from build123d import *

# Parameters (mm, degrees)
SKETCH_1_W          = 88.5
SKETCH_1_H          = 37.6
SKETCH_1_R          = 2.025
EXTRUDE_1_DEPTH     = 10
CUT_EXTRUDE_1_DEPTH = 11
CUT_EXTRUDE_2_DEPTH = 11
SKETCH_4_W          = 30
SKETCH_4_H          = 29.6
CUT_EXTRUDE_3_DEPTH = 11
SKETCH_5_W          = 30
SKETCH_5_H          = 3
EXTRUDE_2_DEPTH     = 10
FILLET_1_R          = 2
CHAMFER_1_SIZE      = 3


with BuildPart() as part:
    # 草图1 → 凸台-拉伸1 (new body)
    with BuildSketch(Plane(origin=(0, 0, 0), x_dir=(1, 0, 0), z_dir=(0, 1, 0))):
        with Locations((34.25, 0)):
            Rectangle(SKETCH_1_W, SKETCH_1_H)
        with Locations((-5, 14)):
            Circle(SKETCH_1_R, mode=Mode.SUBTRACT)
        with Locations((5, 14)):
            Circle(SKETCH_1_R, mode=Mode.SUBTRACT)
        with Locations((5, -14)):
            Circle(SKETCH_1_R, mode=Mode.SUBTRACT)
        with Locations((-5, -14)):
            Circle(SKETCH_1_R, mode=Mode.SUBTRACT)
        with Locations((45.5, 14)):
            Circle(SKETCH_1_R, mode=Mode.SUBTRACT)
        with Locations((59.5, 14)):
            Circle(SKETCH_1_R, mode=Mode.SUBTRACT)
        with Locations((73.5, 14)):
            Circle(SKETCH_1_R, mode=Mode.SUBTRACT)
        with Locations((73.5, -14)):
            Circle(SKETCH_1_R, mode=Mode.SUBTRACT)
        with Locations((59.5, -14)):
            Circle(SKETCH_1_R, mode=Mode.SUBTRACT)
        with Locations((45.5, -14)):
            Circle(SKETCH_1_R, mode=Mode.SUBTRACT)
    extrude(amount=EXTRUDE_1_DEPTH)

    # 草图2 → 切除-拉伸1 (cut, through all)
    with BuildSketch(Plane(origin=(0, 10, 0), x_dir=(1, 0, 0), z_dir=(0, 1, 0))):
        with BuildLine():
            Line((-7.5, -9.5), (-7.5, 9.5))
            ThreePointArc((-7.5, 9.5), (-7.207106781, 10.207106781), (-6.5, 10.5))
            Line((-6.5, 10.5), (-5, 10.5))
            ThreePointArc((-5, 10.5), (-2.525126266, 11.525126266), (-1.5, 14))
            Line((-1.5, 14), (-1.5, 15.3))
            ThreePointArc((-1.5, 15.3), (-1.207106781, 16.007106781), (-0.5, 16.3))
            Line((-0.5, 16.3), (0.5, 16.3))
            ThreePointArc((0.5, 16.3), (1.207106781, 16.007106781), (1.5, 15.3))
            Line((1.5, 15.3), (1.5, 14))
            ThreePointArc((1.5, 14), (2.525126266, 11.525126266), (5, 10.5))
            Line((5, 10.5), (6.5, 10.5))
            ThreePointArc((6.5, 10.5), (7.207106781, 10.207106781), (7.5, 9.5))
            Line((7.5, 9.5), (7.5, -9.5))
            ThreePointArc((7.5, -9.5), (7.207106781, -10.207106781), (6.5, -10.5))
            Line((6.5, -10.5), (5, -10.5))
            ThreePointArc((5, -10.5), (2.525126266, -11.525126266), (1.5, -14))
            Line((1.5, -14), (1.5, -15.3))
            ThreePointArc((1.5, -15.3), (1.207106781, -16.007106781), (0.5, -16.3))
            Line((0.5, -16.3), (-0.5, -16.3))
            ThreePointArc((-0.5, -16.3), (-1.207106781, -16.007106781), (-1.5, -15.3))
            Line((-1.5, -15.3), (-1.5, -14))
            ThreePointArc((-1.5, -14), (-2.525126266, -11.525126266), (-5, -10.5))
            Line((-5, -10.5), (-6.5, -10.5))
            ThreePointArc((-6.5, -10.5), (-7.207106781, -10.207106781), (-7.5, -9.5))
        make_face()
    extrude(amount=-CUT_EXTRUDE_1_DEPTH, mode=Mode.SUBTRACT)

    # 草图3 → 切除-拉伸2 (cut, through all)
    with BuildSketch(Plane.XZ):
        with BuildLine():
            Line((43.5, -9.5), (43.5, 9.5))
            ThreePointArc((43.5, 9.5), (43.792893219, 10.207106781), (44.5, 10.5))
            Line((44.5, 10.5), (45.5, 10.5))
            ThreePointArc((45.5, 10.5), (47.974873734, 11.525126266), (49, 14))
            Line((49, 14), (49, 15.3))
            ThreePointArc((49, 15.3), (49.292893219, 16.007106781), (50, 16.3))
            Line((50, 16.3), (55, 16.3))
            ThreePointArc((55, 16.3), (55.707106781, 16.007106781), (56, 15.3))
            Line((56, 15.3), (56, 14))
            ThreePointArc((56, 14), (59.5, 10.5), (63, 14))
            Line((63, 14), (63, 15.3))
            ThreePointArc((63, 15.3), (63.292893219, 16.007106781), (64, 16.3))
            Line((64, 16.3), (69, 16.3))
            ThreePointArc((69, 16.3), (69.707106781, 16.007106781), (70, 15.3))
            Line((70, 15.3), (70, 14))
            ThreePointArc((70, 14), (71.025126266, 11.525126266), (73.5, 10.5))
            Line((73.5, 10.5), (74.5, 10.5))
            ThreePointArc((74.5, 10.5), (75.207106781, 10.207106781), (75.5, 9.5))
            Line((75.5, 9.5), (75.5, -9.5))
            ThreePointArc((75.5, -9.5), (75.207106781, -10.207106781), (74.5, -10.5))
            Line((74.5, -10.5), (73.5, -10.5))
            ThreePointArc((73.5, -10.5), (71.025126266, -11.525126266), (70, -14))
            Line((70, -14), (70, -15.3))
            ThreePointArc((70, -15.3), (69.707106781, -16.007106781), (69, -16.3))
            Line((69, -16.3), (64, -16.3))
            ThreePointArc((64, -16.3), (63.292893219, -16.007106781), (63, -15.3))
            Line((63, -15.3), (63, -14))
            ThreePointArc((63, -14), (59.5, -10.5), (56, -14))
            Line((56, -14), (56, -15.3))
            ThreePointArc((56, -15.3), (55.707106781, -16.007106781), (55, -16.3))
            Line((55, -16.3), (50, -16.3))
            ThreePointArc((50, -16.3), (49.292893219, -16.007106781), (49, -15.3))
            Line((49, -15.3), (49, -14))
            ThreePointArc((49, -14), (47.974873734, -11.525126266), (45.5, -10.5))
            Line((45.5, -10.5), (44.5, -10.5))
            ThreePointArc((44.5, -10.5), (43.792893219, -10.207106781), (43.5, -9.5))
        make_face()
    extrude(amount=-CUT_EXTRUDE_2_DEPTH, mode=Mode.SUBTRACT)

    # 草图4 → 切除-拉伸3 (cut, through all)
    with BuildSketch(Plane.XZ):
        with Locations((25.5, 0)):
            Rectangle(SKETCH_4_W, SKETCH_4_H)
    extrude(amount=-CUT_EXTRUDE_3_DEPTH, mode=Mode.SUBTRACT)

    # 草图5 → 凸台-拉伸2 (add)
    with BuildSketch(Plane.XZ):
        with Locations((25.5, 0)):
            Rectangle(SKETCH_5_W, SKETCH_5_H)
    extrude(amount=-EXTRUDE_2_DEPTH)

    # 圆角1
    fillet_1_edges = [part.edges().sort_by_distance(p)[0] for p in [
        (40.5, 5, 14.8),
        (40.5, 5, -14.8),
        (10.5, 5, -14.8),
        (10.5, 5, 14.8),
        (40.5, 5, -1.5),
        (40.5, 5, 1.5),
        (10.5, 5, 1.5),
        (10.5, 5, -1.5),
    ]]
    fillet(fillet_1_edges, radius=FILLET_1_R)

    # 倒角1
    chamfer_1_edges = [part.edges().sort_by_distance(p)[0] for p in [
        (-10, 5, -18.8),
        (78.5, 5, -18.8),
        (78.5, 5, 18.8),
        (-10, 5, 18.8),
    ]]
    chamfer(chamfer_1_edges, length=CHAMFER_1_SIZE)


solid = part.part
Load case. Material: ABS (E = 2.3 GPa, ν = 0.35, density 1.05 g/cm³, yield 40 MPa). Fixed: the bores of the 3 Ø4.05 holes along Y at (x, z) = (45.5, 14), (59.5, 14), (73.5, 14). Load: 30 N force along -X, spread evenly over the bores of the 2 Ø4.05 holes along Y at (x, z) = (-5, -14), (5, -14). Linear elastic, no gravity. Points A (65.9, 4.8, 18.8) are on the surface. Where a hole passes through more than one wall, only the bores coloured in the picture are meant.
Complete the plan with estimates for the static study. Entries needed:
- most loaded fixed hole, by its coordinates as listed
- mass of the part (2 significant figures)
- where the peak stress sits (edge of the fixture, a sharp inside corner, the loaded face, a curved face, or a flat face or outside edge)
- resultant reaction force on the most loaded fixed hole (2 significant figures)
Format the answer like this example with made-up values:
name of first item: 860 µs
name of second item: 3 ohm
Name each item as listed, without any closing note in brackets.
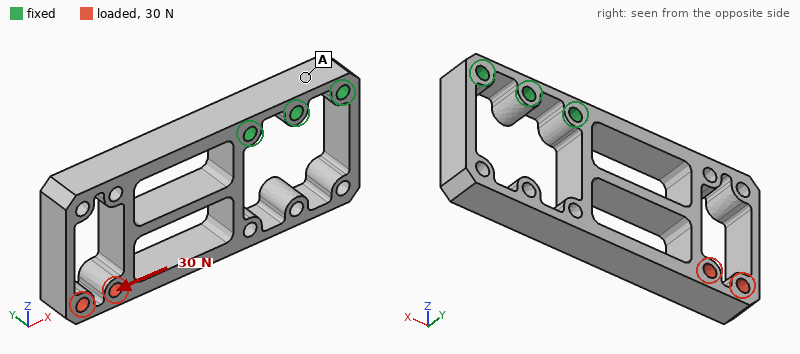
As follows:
most loaded fixed hole, by its coordinates as listed: (45.5, 14)
mass of the part: 12 g
where the peak stress sits: a curved face
resultant reaction force on the most loaded fixed hole: 29 N
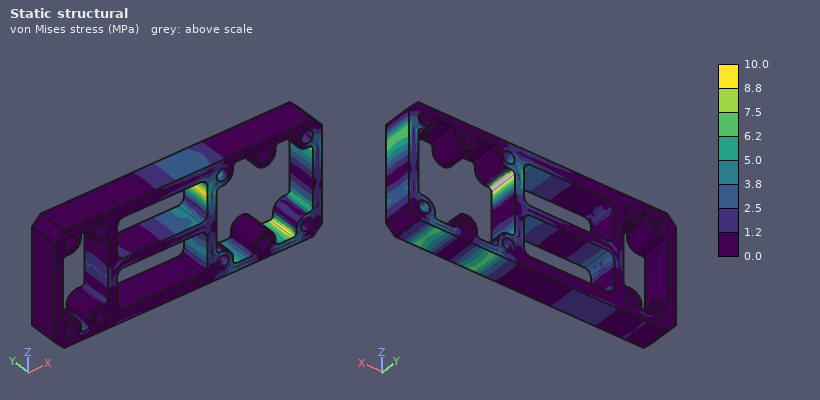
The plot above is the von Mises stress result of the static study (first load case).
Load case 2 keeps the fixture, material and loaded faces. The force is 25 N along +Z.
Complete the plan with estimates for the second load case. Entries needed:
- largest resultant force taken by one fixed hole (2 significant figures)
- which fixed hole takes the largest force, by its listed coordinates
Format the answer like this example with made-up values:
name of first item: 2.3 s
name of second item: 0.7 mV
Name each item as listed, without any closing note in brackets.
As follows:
largest resultant force taken by one fixed hole: 37 N
which fixed hole takes the largest force, by its listed coordinates: (45.5, 14)
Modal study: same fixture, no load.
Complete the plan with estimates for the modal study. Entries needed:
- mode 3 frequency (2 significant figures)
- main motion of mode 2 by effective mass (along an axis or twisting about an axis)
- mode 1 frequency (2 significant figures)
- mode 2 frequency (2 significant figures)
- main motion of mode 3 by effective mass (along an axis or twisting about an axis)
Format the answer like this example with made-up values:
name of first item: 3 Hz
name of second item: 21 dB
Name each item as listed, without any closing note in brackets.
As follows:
mode 3 frequency: 840 Hz
main motion of mode 2 by effective mass: along Y
mode 1 frequency: 370 Hz
mode 2 frequency: 380 Hz
main motion of mode 3 by effective mass: twisting about X
